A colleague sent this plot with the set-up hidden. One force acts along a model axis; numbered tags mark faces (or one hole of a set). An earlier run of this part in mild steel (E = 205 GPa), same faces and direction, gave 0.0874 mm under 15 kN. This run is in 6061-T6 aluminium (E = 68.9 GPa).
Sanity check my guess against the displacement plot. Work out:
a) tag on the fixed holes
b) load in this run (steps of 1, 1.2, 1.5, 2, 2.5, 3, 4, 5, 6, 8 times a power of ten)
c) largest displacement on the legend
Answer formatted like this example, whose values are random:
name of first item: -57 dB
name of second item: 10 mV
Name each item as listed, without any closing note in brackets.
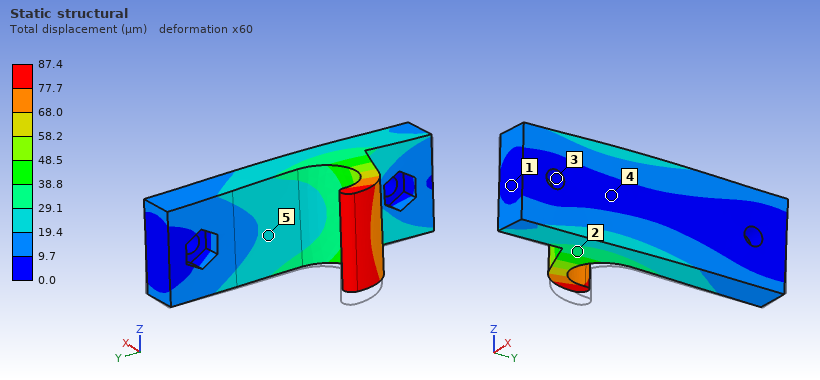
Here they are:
tag on the fixed holes: 3
load in this run: 5 kN
largest displacement on the legend: 87.4 µm
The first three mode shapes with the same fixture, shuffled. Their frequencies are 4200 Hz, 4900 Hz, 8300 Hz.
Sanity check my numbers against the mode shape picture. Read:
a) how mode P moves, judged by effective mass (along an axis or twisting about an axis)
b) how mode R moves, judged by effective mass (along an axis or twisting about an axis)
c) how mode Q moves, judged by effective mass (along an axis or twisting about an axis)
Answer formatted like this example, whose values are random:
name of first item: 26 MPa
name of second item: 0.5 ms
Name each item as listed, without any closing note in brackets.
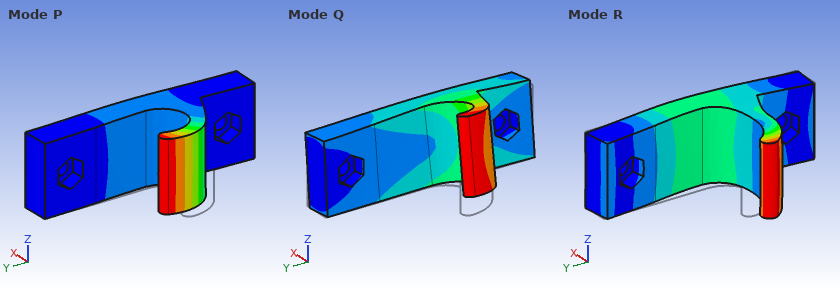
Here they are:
how mode P moves, judged by effective mass: along X
how mode R moves, judged by effective mass: along X
how mode Q moves, judged by effective mass: along Z
